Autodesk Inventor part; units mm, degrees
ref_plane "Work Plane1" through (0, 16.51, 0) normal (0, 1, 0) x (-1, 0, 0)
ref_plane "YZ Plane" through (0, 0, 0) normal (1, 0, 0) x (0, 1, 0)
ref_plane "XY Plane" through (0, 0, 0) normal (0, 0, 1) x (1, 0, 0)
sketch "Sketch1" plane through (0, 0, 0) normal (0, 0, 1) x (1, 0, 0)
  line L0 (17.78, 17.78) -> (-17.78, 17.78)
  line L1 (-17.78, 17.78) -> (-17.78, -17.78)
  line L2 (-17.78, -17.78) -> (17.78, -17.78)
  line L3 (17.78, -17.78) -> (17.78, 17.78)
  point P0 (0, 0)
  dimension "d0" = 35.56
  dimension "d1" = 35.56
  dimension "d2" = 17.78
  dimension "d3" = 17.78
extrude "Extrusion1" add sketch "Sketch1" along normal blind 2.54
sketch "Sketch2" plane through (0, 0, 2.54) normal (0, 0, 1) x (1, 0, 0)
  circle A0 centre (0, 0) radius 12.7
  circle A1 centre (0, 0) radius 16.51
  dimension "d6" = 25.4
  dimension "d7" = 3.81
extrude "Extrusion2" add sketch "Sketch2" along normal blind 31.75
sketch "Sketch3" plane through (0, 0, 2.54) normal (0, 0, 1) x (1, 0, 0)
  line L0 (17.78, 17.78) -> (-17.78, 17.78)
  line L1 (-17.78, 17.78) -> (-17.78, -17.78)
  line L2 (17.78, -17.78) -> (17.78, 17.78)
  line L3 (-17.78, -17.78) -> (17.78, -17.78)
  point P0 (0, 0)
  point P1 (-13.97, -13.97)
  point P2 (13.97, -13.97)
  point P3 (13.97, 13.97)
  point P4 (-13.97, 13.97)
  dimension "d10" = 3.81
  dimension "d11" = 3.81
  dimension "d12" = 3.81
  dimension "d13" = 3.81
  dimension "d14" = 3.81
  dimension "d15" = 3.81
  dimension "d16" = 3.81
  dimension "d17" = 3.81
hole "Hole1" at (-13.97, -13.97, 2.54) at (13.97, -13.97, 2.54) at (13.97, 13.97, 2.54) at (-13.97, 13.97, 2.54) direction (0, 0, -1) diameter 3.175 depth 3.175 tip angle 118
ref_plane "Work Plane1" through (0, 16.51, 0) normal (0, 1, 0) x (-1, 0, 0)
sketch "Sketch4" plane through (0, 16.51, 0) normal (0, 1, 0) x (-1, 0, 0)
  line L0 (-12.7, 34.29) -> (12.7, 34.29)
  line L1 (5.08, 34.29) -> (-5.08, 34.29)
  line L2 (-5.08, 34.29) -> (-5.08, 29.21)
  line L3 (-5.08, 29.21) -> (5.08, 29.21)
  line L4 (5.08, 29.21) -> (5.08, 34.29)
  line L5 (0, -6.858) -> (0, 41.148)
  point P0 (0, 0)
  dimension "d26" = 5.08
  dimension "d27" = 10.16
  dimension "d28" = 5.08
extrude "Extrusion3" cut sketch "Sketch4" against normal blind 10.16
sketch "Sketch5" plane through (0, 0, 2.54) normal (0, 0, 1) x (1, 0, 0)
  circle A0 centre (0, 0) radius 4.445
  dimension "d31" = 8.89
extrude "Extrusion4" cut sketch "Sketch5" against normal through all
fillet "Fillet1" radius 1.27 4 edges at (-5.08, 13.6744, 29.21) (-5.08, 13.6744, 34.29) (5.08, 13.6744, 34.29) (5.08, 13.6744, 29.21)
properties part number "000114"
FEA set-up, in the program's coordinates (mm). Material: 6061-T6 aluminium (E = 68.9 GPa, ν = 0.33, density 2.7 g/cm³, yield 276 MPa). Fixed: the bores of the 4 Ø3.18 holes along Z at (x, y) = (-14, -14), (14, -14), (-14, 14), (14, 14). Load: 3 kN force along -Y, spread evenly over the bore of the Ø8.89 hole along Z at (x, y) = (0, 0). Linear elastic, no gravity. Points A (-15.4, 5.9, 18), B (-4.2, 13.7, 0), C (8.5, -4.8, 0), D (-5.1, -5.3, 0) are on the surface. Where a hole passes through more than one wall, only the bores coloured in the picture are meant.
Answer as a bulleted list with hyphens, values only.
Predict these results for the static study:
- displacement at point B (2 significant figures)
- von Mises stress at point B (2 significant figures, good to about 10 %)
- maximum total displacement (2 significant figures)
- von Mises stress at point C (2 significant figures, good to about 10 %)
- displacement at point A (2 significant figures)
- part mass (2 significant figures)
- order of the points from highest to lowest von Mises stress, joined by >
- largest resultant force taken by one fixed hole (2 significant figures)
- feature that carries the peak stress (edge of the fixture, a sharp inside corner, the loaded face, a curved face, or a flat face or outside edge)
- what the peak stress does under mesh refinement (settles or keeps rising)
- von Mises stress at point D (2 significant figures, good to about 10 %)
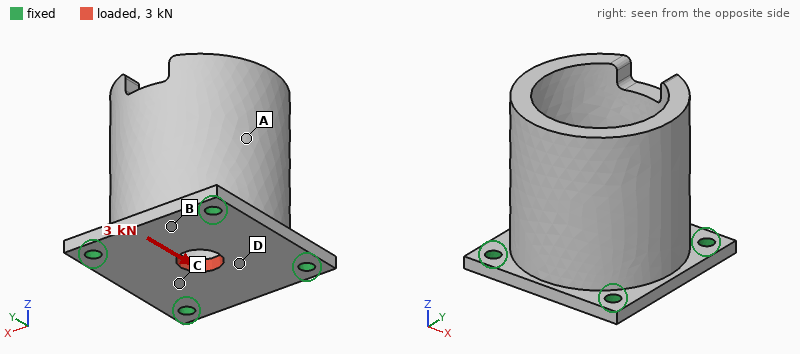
- 7.0 µm
- 18 MPa
- 11 µm
- 27 MPa
- 2.5 µm
- 37 g
- D > C > B > A
- 810 N
- edge of the fixture
- keeps rising
- 33 MPa
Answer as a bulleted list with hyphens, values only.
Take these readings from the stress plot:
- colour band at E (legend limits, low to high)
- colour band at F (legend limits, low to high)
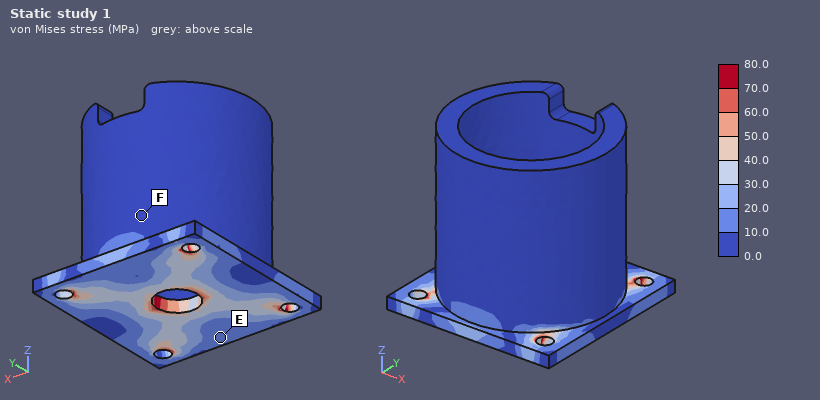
- 10.0 to 20.0 MPa
- 0.0 to 10.0 MPa
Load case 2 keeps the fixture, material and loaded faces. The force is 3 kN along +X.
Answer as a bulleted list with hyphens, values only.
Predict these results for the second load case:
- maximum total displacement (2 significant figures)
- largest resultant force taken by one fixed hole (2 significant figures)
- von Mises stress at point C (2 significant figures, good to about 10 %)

- 11 µm
- 810 N
- 29 MPa
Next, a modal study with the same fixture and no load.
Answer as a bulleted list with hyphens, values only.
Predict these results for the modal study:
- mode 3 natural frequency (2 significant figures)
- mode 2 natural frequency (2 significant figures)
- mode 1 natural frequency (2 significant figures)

- 12 kHz
- 7700 Hz
- 7600 Hz
